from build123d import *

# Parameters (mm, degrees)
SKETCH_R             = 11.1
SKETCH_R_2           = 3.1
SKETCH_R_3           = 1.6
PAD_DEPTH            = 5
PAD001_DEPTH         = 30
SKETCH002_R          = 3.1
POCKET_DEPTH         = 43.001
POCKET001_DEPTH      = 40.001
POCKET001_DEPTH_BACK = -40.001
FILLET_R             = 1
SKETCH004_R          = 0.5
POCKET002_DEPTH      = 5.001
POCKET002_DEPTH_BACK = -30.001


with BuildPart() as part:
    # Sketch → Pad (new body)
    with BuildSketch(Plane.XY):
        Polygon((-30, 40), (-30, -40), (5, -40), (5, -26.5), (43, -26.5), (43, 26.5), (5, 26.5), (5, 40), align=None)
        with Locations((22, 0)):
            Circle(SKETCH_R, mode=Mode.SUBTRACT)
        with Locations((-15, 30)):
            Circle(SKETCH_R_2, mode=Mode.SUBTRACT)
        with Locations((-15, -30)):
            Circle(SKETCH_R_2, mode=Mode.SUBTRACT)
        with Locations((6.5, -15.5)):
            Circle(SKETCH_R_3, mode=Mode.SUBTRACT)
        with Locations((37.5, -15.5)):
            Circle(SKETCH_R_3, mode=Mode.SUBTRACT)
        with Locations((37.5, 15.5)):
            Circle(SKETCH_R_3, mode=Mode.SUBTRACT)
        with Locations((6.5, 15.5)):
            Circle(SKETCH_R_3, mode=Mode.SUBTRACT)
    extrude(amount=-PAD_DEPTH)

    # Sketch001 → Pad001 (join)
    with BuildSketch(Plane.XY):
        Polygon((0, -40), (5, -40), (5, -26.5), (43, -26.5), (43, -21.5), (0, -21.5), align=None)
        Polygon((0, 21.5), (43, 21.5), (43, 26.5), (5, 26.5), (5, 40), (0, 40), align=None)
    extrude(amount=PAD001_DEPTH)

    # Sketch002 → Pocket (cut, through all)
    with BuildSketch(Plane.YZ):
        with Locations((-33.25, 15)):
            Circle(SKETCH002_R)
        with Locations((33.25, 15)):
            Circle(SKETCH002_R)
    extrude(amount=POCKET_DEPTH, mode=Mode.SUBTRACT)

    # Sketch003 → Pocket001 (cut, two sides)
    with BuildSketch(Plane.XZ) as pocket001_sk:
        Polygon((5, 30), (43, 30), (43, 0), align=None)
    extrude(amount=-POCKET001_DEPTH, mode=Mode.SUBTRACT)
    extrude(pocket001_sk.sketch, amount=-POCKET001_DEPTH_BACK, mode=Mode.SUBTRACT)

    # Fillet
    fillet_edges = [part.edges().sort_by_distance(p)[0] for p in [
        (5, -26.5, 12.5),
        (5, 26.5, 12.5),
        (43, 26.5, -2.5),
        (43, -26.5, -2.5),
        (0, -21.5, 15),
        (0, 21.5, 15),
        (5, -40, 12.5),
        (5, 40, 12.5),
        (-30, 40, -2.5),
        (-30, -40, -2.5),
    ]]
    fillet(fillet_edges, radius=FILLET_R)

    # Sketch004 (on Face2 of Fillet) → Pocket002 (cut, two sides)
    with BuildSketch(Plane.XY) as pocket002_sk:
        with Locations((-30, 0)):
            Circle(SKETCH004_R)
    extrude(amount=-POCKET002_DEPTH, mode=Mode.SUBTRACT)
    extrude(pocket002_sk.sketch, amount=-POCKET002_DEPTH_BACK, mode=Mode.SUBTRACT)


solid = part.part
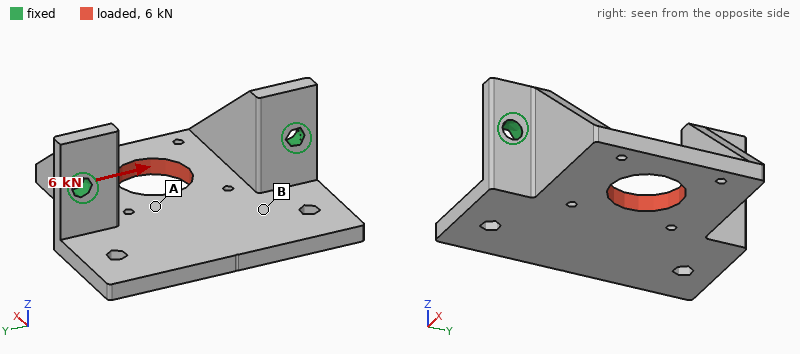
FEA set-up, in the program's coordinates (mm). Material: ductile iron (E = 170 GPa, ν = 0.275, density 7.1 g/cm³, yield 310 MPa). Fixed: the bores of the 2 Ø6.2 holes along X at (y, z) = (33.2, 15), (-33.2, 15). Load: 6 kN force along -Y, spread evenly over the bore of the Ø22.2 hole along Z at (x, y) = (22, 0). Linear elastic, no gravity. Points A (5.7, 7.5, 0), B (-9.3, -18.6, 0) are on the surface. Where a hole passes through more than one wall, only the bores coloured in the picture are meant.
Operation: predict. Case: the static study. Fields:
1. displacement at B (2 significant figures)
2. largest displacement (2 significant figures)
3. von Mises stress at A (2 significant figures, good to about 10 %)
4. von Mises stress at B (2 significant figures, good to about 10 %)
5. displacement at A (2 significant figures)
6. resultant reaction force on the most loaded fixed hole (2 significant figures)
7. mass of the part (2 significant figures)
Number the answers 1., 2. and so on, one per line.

1. 17 µm
2. 91 µm
3. 74 MPa
4. 28 MPa
5. 30 µm
6. 3.5 kN
7. 230 g
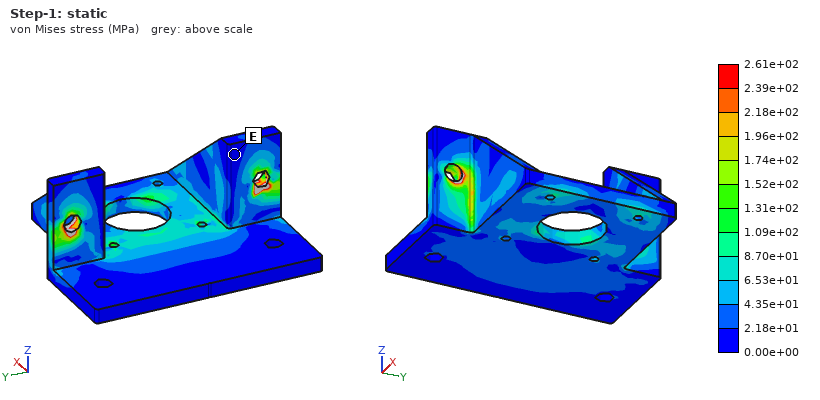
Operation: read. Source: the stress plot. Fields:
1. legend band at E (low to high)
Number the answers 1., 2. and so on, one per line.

1. 0.00e+00 to 2.18e+01 MPa
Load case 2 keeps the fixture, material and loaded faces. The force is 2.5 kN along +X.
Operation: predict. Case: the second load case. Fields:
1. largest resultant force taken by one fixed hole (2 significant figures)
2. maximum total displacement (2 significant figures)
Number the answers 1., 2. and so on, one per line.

1. 1.3 kN
2. 80 µm
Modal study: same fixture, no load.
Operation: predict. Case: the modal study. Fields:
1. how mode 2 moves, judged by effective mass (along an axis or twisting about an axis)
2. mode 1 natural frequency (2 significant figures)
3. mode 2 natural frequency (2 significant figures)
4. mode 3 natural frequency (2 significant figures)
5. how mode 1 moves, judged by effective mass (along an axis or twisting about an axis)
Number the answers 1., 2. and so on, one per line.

1. twisting about Z
2. 1900 Hz
3. 3400 Hz
4. 3700 Hz
5. along X
